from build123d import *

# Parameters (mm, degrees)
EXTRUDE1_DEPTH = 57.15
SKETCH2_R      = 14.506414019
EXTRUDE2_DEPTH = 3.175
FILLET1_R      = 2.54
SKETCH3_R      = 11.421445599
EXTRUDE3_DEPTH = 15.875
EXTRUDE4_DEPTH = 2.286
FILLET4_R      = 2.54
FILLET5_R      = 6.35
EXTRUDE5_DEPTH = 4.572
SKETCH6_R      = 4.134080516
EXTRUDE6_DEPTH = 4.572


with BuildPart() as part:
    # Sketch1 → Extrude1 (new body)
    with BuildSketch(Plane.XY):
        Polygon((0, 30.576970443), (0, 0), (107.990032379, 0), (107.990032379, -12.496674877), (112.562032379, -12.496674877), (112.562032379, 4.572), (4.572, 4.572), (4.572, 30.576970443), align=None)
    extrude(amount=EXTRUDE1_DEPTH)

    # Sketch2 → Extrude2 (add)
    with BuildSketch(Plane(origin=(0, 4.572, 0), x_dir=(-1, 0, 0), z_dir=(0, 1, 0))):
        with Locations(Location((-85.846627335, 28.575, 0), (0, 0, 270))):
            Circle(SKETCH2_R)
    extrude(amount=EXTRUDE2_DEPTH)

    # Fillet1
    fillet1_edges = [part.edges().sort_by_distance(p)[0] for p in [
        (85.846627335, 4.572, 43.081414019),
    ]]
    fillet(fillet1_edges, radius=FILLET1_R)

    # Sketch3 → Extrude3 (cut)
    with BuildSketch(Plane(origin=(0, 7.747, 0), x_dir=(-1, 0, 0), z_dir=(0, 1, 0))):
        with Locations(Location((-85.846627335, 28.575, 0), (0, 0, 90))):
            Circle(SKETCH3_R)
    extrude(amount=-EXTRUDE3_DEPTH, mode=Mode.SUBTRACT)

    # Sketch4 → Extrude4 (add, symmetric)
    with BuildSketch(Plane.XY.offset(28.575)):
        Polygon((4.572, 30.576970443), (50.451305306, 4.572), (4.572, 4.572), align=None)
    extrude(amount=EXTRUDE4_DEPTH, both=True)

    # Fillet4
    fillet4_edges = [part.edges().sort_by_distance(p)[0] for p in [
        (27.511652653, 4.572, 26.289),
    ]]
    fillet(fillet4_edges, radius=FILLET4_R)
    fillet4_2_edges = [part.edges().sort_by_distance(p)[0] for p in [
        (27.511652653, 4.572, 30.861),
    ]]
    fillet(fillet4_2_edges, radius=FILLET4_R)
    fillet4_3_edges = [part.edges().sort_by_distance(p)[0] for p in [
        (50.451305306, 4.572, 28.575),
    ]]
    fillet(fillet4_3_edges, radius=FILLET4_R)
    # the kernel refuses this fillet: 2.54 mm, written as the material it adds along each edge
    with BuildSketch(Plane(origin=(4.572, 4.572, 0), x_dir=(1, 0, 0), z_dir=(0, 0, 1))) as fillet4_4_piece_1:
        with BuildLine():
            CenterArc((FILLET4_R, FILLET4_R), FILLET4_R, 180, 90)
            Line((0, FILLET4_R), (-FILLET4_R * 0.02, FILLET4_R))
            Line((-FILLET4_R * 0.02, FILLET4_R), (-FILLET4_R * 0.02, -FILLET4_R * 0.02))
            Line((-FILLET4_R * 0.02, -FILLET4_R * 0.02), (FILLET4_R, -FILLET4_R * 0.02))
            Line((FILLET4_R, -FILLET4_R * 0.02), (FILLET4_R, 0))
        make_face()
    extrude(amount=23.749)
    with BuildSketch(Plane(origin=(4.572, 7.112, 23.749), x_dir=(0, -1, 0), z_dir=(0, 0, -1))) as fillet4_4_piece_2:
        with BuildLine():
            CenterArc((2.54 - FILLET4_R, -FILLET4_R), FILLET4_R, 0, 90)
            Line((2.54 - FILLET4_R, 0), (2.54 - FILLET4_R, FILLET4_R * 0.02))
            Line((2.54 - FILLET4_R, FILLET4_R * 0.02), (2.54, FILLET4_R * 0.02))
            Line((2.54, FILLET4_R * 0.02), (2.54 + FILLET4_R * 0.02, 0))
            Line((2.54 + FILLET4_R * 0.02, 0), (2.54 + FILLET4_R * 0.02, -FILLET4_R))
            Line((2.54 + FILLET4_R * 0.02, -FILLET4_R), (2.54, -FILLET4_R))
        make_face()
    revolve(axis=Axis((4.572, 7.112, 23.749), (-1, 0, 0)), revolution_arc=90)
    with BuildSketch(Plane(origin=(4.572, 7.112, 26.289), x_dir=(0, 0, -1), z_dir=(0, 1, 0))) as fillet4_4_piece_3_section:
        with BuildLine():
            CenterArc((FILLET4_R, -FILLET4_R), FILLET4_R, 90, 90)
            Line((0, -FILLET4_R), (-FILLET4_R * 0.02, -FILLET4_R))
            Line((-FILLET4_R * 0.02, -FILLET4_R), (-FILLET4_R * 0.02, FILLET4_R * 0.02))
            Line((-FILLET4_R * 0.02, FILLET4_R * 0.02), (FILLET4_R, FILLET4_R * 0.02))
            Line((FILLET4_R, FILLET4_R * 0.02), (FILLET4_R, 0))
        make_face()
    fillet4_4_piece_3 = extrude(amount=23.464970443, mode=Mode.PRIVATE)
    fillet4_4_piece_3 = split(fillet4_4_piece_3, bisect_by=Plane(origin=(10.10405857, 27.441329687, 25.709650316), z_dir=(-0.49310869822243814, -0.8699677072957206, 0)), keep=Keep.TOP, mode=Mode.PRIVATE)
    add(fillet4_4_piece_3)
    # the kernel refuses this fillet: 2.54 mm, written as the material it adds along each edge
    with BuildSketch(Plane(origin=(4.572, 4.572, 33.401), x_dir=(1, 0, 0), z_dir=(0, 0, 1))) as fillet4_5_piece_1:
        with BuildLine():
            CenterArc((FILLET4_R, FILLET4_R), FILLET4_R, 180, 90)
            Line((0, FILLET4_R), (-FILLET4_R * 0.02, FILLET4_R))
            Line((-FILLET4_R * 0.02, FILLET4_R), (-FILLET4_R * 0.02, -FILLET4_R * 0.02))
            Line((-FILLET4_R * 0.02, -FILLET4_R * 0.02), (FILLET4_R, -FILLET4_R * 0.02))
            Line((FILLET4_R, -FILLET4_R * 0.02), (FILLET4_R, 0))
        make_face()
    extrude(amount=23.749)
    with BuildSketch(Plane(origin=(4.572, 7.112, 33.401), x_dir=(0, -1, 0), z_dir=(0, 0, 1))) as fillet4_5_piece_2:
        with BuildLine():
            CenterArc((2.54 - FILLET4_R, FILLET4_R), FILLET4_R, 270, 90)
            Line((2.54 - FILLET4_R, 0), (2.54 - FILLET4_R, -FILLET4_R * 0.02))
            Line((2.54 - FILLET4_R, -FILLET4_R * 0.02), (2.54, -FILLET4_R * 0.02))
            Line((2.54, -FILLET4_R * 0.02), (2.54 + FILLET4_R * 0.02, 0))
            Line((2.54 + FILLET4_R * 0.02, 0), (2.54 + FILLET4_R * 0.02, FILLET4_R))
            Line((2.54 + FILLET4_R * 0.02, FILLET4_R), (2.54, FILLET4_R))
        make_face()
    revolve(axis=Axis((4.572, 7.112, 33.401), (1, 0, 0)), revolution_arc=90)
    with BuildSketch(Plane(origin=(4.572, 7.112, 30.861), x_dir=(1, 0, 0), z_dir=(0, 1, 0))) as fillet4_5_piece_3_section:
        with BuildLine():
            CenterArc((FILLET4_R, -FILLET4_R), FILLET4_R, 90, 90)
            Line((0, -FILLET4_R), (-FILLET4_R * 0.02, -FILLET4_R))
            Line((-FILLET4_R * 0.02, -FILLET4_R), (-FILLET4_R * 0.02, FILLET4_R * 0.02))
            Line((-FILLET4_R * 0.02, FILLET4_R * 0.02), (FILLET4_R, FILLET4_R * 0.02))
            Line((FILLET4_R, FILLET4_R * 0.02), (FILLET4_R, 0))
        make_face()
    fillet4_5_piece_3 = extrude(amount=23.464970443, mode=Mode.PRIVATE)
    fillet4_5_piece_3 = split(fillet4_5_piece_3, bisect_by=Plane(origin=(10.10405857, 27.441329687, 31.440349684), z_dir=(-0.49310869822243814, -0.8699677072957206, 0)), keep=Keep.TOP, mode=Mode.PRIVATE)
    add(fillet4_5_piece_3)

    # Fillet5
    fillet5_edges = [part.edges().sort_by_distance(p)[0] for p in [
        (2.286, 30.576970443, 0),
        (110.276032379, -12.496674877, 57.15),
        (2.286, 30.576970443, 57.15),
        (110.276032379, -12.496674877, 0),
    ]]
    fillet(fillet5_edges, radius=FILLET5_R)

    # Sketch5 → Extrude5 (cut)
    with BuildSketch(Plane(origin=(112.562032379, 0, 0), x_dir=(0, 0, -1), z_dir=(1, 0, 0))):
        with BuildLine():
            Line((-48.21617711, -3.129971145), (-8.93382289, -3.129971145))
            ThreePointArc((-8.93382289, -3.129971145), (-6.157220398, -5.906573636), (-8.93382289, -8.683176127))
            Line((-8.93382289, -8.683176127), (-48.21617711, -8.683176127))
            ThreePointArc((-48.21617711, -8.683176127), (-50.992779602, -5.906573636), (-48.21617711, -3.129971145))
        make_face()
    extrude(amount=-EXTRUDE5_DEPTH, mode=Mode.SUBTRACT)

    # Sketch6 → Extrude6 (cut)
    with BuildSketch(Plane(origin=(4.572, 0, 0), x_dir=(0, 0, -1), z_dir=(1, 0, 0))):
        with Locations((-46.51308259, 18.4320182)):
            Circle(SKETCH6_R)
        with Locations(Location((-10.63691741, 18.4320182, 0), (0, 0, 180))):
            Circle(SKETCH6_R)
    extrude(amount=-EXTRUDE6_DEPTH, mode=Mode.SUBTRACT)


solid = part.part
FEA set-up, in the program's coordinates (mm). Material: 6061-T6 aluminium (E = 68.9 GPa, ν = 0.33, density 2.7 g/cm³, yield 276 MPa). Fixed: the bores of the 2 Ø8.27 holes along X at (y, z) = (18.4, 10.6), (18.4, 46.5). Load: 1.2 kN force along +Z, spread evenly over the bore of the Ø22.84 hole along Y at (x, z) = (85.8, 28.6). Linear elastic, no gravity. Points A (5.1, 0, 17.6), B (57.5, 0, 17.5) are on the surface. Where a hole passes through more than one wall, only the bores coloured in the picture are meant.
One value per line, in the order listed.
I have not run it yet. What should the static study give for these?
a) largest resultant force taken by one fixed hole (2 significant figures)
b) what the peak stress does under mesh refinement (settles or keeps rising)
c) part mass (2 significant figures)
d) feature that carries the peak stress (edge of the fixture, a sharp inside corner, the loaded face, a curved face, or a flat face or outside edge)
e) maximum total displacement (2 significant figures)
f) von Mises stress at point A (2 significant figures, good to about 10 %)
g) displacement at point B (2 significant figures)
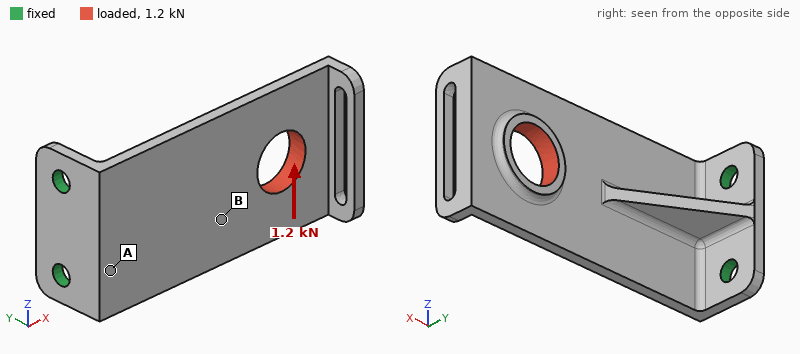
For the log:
2.8 kN
keeps rising
110 g
edge of the fixture
0.61 mm
75 MPa
0.27 mm
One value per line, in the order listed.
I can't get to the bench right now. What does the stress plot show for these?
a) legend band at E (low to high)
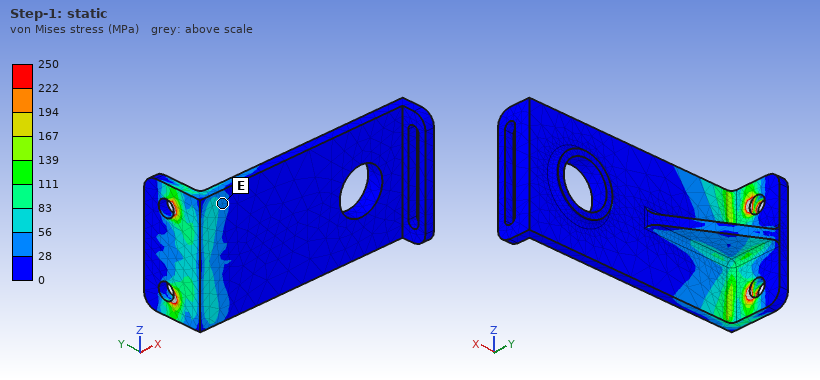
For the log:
28 to 56 MPa
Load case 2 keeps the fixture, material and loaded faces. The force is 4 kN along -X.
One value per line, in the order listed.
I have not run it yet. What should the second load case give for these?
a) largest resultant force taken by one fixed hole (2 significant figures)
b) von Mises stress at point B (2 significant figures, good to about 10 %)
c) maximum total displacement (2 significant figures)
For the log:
2.0 kN
15 MPa
0.29 mm
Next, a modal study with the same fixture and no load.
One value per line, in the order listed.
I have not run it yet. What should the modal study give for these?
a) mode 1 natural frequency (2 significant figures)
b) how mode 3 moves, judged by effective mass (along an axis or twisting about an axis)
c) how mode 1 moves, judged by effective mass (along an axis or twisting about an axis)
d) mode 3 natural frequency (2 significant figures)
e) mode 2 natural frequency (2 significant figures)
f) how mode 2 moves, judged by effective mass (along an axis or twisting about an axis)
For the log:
460 Hz
along Z
along Y
1200 Hz
1100 Hz
along Z
